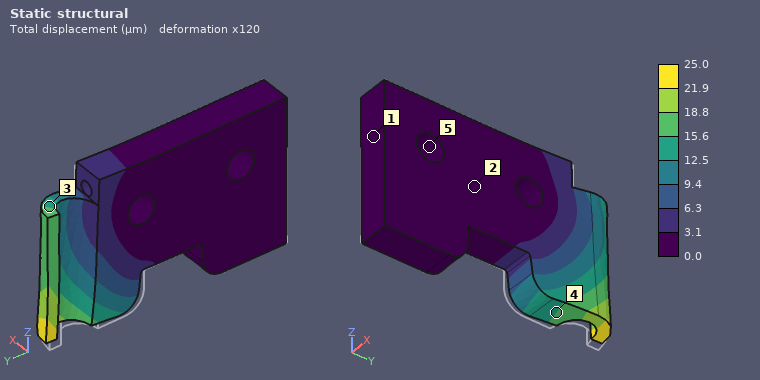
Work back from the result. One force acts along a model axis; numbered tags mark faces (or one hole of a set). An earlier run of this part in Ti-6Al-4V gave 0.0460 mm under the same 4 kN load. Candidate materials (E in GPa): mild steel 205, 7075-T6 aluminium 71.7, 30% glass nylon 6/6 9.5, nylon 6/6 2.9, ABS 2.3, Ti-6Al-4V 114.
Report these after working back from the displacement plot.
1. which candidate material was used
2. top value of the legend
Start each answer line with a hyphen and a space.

- mild steel
- 25.0 µm
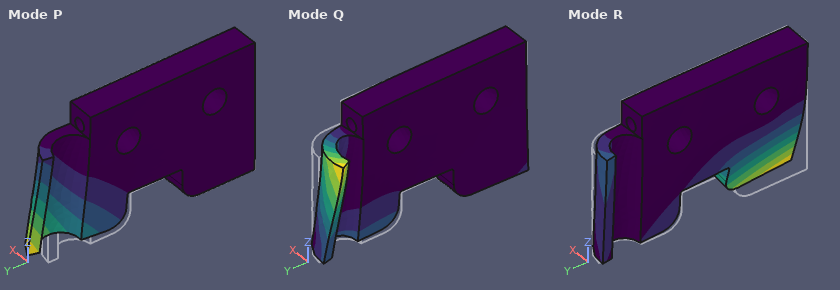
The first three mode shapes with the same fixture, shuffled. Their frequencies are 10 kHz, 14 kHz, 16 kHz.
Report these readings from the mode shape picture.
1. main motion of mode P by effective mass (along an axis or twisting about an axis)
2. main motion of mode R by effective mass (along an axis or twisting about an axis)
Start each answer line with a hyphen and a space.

- along X
- along X
